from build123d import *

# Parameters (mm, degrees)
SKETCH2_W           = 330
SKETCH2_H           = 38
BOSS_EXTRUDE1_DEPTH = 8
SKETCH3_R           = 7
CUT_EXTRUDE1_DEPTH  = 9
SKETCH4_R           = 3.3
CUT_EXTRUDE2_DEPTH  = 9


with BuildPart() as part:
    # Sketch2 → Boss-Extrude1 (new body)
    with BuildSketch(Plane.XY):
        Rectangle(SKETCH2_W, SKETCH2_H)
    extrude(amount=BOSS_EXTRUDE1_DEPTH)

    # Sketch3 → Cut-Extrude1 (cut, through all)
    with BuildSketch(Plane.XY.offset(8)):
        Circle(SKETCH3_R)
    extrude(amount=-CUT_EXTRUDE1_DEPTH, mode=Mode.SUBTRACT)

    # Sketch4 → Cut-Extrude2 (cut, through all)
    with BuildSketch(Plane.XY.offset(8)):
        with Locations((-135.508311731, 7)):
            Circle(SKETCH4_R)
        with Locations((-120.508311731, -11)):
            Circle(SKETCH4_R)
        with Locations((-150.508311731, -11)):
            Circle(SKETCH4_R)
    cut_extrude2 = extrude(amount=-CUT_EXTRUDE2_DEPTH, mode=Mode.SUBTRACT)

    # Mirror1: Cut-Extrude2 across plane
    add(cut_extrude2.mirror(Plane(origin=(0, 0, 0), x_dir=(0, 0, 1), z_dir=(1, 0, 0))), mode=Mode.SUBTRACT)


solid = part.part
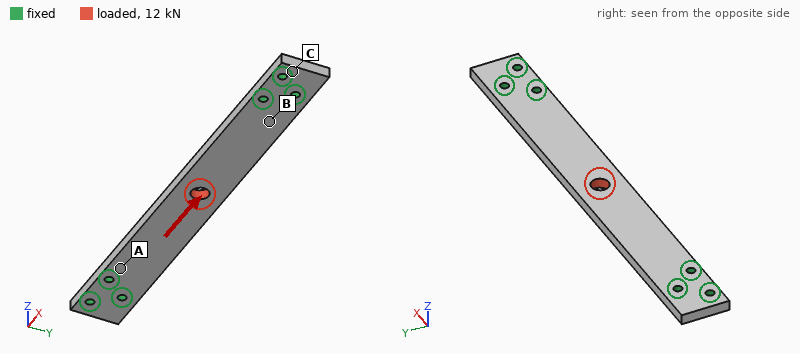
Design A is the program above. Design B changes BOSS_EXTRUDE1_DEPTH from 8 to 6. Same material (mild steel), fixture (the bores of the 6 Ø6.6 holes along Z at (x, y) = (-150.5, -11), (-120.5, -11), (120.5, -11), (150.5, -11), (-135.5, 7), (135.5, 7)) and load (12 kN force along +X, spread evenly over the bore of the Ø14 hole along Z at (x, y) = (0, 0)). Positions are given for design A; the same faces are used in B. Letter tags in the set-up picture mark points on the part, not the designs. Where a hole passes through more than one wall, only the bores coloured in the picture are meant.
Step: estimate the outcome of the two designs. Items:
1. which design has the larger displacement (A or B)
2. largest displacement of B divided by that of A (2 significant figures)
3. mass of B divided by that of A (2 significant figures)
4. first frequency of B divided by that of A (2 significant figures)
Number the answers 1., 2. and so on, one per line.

1. B
2. 1.3
3. 0.75
4. 0.76
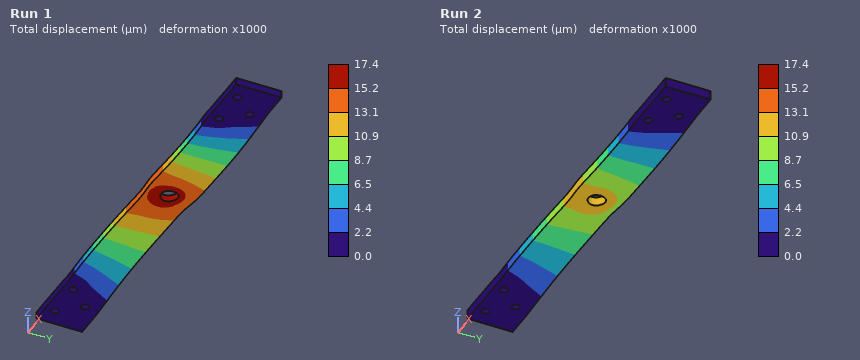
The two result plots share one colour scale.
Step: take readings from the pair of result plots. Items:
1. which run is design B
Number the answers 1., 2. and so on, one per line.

1. Run 1
